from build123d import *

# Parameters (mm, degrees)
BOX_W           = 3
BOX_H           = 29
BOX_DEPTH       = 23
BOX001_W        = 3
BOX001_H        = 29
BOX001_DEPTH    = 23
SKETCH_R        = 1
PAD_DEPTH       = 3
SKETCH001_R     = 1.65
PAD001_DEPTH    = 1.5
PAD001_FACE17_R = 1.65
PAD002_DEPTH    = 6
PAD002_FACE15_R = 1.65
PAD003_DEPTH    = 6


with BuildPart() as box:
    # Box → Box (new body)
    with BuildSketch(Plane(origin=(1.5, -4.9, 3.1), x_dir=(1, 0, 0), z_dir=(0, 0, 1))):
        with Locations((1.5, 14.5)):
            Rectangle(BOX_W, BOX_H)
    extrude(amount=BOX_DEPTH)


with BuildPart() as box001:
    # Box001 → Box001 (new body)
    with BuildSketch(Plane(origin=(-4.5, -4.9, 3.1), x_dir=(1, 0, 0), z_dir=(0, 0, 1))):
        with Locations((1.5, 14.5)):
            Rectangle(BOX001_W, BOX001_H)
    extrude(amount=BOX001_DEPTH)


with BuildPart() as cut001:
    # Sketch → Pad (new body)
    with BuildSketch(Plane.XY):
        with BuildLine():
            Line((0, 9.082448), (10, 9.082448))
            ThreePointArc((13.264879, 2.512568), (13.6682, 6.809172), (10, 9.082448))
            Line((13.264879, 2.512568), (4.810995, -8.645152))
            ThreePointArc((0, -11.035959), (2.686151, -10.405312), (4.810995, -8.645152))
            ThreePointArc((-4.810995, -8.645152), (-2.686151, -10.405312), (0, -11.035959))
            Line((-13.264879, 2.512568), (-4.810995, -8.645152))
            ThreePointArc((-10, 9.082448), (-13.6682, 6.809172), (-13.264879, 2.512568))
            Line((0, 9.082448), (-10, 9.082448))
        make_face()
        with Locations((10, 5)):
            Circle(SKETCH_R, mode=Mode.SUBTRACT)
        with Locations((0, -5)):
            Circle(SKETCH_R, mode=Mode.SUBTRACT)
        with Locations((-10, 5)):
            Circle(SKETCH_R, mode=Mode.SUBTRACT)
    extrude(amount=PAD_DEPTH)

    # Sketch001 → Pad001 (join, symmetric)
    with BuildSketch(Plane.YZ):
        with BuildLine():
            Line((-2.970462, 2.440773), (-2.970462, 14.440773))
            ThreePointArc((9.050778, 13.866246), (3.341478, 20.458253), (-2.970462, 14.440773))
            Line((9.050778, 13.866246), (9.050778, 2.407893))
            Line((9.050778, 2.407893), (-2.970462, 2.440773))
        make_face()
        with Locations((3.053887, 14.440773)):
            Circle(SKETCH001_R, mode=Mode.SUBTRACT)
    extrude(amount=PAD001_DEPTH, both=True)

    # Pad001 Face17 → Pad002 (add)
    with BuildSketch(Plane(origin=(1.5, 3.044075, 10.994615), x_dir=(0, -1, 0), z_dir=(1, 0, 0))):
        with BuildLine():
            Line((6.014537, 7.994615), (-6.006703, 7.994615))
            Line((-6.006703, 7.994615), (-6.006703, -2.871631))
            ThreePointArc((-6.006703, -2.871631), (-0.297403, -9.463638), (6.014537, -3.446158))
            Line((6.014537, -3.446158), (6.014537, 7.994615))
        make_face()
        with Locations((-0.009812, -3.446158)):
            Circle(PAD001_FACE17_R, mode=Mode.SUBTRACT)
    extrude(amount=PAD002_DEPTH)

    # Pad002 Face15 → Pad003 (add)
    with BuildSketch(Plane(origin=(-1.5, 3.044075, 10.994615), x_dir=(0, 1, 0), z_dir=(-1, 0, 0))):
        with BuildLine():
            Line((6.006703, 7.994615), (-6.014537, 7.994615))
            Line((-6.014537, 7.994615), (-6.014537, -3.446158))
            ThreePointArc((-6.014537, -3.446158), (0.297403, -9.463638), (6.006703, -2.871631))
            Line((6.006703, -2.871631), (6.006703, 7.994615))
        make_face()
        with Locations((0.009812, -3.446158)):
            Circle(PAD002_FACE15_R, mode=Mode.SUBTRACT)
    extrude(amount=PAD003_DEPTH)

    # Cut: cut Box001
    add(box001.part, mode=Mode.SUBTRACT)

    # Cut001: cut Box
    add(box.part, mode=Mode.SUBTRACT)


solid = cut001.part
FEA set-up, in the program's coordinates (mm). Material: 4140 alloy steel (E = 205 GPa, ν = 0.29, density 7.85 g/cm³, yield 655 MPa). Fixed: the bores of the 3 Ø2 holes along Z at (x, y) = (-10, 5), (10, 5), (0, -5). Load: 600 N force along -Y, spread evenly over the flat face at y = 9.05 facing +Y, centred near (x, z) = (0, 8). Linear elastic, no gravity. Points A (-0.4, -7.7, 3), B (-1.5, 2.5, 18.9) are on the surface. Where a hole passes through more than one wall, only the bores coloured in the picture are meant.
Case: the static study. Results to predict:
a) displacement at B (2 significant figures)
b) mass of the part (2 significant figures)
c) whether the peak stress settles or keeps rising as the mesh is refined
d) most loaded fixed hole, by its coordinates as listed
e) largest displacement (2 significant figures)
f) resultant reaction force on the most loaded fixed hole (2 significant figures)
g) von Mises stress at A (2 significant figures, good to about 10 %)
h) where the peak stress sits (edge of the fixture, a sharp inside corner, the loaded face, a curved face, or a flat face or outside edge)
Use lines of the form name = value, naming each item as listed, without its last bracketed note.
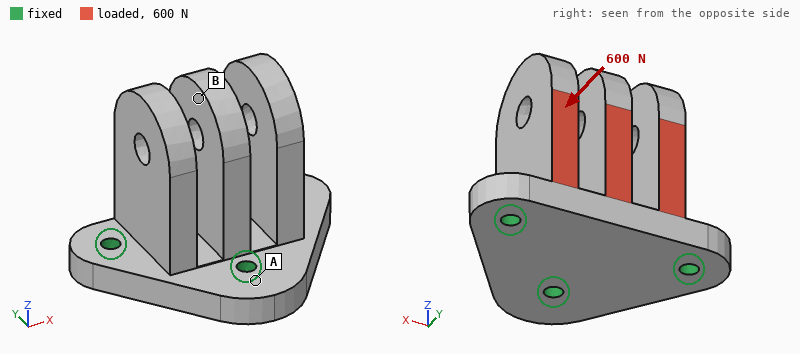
displacement at B = 7.8 µm
mass of the part = 22 g
whether the peak stress settles or keeps rising as the mesh is refined = keeps rising
most loaded fixed hole, by its coordinates as listed = (0, -5)
largest displacement = 9.1 µm
resultant reaction force on the most loaded fixed hole = 430 N
von Mises stress at A = 16 MPa
where the peak stress sits = edge of the fixture
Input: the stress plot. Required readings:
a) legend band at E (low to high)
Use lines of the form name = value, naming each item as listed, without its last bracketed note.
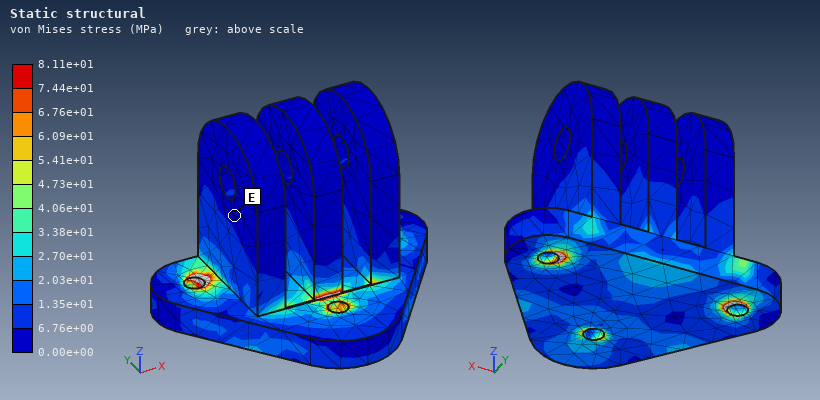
legend band at E = 0.00e+00 to 6.76e+00 MPa
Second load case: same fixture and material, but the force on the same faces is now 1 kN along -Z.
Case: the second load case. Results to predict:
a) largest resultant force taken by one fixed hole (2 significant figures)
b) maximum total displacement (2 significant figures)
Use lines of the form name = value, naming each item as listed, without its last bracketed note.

largest resultant force taken by one fixed hole = 570 N
maximum total displacement = 20 µm
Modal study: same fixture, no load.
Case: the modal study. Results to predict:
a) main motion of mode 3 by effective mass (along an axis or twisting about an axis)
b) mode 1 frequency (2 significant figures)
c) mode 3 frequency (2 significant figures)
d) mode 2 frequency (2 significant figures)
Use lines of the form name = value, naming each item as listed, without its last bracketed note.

main motion of mode 3 by effective mass = along X
mode 1 frequency = 7200 Hz
mode 3 frequency = 8400 Hz
mode 2 frequency = 7800 Hz
